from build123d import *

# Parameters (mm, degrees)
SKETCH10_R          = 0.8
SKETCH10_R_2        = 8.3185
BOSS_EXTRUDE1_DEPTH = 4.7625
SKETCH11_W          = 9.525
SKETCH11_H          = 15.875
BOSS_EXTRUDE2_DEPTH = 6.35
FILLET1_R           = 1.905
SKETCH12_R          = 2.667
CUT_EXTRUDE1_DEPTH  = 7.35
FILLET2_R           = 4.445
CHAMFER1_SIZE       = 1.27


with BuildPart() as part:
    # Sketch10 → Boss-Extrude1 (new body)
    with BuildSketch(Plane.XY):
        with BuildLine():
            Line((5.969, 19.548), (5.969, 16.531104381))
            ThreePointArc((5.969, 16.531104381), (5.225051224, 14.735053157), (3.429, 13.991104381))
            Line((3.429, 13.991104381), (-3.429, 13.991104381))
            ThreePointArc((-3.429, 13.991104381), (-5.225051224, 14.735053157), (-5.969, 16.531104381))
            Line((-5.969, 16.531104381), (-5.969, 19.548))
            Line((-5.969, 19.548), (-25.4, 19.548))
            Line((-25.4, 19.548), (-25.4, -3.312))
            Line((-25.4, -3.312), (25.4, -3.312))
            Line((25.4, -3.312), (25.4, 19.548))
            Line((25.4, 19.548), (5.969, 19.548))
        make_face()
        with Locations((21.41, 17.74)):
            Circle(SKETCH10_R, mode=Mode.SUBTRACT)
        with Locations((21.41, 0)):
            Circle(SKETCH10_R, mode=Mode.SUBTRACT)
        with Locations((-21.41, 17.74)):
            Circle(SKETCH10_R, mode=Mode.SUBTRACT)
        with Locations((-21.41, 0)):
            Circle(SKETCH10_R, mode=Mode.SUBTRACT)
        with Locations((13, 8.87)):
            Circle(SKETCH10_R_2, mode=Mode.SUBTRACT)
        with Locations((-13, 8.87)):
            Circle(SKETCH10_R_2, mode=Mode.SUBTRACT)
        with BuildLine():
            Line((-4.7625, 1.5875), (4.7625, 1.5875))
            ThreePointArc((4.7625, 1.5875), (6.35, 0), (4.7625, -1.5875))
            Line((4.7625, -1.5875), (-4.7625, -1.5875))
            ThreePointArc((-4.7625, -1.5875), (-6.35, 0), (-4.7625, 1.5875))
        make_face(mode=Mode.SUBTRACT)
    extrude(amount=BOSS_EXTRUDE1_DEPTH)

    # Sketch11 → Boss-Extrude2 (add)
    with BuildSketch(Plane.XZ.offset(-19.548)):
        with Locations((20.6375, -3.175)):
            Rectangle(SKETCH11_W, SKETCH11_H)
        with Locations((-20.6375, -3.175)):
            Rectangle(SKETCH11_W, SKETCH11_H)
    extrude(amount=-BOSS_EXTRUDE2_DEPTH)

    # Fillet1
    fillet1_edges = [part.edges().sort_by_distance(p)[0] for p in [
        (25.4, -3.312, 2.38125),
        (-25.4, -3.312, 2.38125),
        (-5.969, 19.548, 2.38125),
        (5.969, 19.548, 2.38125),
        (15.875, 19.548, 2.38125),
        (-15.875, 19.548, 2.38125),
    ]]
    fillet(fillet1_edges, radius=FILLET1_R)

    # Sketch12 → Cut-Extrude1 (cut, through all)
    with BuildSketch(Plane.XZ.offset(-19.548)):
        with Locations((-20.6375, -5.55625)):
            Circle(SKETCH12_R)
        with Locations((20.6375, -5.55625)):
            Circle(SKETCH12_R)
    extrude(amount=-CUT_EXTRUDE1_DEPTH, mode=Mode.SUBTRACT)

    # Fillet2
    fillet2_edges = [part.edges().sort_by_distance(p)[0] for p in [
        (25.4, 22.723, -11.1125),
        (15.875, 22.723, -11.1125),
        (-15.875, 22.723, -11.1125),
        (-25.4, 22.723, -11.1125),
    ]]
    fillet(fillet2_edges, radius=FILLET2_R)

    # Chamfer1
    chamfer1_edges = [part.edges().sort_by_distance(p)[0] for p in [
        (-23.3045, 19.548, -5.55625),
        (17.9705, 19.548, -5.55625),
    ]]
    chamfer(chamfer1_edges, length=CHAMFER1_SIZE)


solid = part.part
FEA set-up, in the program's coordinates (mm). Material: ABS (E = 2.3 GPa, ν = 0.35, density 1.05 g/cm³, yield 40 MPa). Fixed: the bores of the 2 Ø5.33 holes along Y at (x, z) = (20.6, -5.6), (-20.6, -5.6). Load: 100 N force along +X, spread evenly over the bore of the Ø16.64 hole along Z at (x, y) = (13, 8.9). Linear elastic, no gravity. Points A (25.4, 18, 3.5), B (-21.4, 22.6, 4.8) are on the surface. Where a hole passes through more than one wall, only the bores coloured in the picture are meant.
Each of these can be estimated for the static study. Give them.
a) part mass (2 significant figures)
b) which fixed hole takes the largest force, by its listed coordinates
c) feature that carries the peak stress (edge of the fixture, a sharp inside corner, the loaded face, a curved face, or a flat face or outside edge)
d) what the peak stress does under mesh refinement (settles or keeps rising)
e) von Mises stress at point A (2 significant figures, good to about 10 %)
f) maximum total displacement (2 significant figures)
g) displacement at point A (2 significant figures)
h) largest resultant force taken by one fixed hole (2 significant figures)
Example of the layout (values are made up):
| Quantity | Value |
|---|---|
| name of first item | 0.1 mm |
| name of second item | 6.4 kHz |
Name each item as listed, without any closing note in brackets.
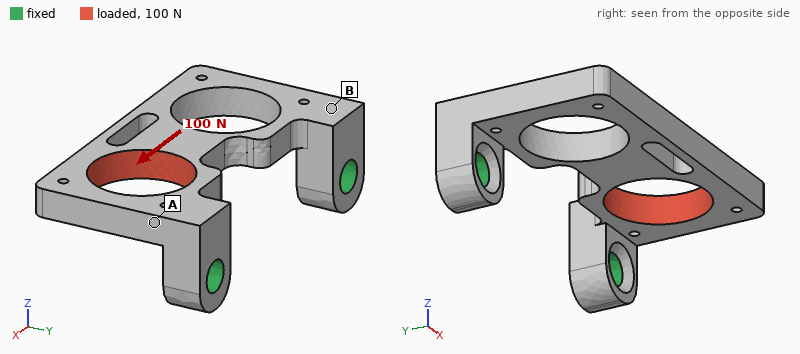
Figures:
| Quantity | Value |
|---|---|
| part mass | 4.6 g |
| which fixed hole takes the largest force, by its listed coordinates | (20.6, -5.6) |
| feature that carries the peak stress | edge of the fixture |
| what the peak stress does under mesh refinement | keeps rising |
| von Mises stress at point A | 2.2 MPa |
| maximum total displacement | 0.12 mm |
| displacement at point A | 0.053 mm |
| largest resultant force taken by one fixed hole | 72 N |
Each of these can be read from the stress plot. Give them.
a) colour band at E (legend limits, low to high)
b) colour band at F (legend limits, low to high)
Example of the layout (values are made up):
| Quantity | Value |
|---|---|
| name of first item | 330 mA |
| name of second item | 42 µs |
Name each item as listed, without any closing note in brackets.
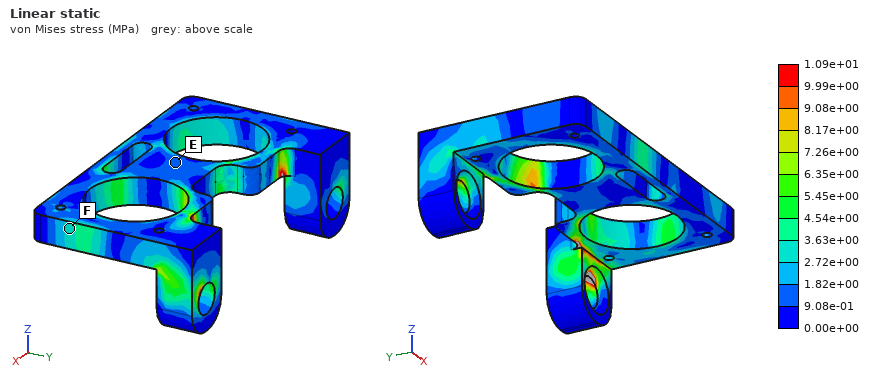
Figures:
| Quantity | Value |
|---|---|
| colour band at E | 9.08e-01 to 1.82e+00 MPa |
| colour band at F | 2.72e+00 to 3.63e+00 MPa |
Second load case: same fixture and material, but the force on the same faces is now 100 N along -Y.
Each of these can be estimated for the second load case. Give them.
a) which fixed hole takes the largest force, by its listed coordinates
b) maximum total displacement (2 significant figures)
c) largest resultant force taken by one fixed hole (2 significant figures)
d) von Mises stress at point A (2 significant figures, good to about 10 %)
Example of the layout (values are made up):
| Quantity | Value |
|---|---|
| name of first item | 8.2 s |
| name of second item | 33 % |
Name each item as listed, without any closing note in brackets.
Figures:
| Quantity | Value |
|---|---|
| which fixed hole takes the largest force, by its listed coordinates | (20.6, -5.6) |
| maximum total displacement | 0.17 mm |
| largest resultant force taken by one fixed hole | 83 N |
| von Mises stress at point A | 3.2 MPa |
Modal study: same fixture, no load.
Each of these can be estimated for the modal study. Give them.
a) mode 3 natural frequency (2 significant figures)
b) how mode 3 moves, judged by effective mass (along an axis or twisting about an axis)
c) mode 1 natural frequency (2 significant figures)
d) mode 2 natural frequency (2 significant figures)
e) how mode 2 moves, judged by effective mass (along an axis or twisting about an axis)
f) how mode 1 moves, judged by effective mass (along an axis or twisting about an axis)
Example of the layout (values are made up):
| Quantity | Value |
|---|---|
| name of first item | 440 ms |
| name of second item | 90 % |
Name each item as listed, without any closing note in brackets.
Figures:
| Quantity | Value |
|---|---|
| mode 3 natural frequency | 2800 Hz |
| how mode 3 moves, judged by effective mass | along X |
| mode 1 natural frequency | 920 Hz |
| mode 2 natural frequency | 1800 Hz |
| how mode 2 moves, judged by effective mass | twisting about Y |
| how mode 1 moves, judged by effective mass | along Z |
